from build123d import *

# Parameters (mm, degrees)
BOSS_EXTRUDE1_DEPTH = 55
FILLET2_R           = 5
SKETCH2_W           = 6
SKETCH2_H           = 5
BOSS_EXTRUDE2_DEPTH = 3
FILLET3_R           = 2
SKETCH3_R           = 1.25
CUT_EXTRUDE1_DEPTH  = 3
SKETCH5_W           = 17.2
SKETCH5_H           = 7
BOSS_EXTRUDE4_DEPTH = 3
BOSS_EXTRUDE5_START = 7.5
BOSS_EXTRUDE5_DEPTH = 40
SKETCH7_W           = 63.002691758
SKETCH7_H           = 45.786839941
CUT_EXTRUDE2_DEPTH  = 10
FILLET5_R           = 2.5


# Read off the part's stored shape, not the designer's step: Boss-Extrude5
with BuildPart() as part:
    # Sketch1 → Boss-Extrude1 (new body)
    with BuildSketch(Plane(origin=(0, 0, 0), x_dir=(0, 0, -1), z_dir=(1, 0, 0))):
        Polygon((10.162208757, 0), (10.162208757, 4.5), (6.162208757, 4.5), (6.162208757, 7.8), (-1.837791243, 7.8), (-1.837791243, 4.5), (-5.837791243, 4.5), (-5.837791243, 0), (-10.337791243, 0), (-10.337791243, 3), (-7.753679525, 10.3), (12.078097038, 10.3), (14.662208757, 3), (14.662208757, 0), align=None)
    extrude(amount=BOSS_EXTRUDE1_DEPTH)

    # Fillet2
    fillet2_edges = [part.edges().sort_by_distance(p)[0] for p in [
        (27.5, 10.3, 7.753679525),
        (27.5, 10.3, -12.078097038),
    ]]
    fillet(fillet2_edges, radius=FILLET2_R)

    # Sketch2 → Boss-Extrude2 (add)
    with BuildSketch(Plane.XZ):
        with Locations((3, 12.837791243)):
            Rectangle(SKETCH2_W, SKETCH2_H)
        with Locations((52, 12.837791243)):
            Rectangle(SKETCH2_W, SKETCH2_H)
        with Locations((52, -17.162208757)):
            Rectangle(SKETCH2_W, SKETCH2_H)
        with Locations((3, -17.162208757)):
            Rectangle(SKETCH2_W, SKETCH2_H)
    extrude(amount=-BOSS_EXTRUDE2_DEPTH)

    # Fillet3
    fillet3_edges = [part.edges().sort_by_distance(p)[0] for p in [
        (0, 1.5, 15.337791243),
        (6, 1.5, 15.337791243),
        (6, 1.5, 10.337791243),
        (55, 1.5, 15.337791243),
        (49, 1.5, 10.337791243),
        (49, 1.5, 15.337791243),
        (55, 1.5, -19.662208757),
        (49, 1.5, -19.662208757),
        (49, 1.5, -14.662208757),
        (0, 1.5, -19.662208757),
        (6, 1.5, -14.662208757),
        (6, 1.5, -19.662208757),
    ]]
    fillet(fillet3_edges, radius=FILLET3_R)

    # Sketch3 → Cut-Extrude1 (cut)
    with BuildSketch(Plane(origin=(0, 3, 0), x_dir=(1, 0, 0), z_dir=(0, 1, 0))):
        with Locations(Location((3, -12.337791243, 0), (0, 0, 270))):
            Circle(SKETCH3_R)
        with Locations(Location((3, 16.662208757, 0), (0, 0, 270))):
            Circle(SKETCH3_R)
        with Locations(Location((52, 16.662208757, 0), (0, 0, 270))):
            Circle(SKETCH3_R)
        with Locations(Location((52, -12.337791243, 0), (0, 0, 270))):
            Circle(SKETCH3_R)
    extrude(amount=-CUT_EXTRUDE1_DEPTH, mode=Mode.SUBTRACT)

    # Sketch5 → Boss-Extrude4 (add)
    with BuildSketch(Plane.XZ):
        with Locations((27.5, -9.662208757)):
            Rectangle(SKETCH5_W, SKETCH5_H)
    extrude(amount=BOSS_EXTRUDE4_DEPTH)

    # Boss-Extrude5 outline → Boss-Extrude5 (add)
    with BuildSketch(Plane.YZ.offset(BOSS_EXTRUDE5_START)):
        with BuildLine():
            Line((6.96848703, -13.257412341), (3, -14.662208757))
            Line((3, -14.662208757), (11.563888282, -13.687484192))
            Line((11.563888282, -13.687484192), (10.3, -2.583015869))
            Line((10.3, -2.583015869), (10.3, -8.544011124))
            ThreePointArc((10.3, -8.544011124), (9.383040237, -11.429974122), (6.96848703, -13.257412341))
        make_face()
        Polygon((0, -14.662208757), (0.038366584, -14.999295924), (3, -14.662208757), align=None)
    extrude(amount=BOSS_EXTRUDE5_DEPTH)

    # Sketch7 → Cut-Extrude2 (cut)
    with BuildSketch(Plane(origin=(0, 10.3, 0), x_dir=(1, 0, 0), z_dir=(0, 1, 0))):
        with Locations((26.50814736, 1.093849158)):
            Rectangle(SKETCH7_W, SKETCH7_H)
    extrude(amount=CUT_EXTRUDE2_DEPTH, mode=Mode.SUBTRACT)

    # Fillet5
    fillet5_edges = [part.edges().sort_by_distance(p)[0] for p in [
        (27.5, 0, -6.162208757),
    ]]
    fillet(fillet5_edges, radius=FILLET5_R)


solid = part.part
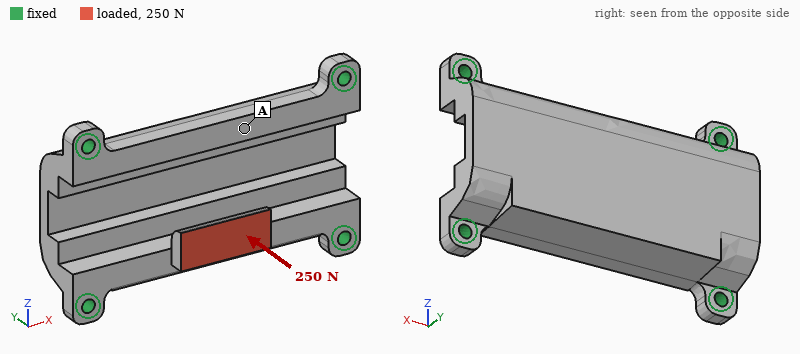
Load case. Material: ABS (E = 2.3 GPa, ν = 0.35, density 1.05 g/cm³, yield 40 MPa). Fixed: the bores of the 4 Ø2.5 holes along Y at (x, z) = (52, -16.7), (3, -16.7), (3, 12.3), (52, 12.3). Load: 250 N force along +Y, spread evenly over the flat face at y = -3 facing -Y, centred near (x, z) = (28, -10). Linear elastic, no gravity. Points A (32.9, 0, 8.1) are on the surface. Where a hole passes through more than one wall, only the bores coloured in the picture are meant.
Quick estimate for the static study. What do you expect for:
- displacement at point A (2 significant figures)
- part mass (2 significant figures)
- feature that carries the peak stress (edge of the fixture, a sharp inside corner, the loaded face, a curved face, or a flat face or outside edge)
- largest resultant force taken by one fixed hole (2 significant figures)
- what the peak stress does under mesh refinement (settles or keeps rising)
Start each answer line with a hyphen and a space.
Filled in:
- 0.081 mm
- 8.9 g
- edge of the fixture
- 130 N
- keeps rising
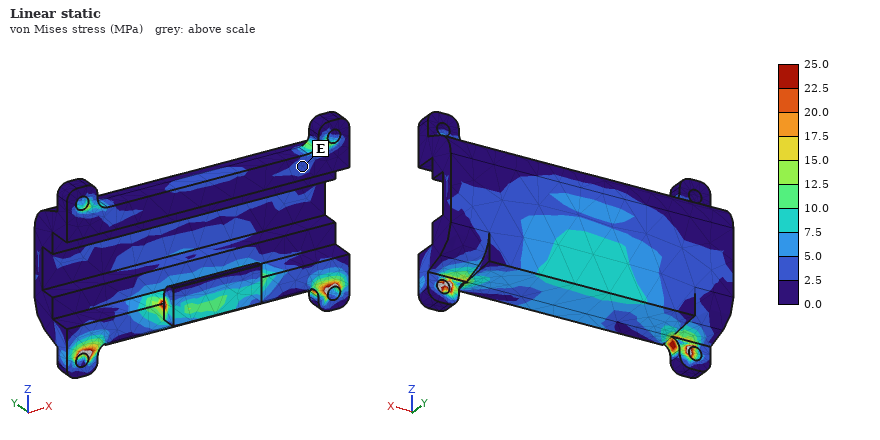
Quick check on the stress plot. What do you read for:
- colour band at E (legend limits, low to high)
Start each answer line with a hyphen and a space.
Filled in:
- 2.5 to 5.0 MPa
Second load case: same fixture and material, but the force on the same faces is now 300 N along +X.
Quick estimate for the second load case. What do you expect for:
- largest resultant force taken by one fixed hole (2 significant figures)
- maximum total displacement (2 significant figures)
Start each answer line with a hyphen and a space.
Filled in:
- 110 N
- 0.18 mm
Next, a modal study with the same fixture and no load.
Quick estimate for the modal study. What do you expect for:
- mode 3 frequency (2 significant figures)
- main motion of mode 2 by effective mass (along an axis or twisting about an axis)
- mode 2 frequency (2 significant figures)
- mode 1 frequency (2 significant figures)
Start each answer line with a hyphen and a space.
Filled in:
- 4700 Hz
- along Y
- 3100 Hz
- 3000 Hz
